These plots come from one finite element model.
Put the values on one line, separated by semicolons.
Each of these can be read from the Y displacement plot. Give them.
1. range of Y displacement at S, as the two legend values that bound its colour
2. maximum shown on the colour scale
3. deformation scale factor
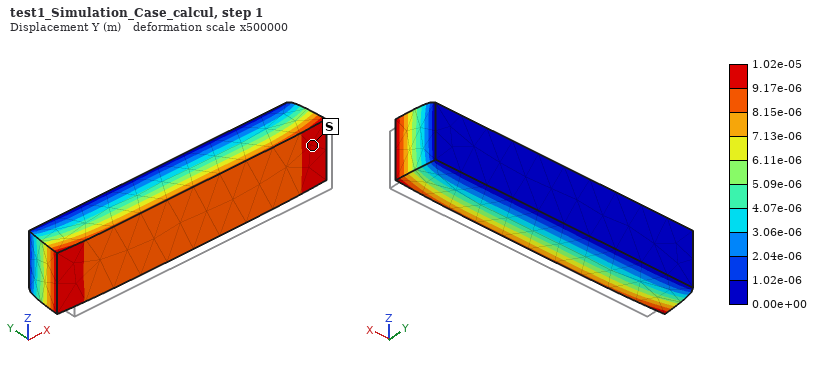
9.17e-06 to 1.02e-05 m; 1.02e-05 m; 500000
